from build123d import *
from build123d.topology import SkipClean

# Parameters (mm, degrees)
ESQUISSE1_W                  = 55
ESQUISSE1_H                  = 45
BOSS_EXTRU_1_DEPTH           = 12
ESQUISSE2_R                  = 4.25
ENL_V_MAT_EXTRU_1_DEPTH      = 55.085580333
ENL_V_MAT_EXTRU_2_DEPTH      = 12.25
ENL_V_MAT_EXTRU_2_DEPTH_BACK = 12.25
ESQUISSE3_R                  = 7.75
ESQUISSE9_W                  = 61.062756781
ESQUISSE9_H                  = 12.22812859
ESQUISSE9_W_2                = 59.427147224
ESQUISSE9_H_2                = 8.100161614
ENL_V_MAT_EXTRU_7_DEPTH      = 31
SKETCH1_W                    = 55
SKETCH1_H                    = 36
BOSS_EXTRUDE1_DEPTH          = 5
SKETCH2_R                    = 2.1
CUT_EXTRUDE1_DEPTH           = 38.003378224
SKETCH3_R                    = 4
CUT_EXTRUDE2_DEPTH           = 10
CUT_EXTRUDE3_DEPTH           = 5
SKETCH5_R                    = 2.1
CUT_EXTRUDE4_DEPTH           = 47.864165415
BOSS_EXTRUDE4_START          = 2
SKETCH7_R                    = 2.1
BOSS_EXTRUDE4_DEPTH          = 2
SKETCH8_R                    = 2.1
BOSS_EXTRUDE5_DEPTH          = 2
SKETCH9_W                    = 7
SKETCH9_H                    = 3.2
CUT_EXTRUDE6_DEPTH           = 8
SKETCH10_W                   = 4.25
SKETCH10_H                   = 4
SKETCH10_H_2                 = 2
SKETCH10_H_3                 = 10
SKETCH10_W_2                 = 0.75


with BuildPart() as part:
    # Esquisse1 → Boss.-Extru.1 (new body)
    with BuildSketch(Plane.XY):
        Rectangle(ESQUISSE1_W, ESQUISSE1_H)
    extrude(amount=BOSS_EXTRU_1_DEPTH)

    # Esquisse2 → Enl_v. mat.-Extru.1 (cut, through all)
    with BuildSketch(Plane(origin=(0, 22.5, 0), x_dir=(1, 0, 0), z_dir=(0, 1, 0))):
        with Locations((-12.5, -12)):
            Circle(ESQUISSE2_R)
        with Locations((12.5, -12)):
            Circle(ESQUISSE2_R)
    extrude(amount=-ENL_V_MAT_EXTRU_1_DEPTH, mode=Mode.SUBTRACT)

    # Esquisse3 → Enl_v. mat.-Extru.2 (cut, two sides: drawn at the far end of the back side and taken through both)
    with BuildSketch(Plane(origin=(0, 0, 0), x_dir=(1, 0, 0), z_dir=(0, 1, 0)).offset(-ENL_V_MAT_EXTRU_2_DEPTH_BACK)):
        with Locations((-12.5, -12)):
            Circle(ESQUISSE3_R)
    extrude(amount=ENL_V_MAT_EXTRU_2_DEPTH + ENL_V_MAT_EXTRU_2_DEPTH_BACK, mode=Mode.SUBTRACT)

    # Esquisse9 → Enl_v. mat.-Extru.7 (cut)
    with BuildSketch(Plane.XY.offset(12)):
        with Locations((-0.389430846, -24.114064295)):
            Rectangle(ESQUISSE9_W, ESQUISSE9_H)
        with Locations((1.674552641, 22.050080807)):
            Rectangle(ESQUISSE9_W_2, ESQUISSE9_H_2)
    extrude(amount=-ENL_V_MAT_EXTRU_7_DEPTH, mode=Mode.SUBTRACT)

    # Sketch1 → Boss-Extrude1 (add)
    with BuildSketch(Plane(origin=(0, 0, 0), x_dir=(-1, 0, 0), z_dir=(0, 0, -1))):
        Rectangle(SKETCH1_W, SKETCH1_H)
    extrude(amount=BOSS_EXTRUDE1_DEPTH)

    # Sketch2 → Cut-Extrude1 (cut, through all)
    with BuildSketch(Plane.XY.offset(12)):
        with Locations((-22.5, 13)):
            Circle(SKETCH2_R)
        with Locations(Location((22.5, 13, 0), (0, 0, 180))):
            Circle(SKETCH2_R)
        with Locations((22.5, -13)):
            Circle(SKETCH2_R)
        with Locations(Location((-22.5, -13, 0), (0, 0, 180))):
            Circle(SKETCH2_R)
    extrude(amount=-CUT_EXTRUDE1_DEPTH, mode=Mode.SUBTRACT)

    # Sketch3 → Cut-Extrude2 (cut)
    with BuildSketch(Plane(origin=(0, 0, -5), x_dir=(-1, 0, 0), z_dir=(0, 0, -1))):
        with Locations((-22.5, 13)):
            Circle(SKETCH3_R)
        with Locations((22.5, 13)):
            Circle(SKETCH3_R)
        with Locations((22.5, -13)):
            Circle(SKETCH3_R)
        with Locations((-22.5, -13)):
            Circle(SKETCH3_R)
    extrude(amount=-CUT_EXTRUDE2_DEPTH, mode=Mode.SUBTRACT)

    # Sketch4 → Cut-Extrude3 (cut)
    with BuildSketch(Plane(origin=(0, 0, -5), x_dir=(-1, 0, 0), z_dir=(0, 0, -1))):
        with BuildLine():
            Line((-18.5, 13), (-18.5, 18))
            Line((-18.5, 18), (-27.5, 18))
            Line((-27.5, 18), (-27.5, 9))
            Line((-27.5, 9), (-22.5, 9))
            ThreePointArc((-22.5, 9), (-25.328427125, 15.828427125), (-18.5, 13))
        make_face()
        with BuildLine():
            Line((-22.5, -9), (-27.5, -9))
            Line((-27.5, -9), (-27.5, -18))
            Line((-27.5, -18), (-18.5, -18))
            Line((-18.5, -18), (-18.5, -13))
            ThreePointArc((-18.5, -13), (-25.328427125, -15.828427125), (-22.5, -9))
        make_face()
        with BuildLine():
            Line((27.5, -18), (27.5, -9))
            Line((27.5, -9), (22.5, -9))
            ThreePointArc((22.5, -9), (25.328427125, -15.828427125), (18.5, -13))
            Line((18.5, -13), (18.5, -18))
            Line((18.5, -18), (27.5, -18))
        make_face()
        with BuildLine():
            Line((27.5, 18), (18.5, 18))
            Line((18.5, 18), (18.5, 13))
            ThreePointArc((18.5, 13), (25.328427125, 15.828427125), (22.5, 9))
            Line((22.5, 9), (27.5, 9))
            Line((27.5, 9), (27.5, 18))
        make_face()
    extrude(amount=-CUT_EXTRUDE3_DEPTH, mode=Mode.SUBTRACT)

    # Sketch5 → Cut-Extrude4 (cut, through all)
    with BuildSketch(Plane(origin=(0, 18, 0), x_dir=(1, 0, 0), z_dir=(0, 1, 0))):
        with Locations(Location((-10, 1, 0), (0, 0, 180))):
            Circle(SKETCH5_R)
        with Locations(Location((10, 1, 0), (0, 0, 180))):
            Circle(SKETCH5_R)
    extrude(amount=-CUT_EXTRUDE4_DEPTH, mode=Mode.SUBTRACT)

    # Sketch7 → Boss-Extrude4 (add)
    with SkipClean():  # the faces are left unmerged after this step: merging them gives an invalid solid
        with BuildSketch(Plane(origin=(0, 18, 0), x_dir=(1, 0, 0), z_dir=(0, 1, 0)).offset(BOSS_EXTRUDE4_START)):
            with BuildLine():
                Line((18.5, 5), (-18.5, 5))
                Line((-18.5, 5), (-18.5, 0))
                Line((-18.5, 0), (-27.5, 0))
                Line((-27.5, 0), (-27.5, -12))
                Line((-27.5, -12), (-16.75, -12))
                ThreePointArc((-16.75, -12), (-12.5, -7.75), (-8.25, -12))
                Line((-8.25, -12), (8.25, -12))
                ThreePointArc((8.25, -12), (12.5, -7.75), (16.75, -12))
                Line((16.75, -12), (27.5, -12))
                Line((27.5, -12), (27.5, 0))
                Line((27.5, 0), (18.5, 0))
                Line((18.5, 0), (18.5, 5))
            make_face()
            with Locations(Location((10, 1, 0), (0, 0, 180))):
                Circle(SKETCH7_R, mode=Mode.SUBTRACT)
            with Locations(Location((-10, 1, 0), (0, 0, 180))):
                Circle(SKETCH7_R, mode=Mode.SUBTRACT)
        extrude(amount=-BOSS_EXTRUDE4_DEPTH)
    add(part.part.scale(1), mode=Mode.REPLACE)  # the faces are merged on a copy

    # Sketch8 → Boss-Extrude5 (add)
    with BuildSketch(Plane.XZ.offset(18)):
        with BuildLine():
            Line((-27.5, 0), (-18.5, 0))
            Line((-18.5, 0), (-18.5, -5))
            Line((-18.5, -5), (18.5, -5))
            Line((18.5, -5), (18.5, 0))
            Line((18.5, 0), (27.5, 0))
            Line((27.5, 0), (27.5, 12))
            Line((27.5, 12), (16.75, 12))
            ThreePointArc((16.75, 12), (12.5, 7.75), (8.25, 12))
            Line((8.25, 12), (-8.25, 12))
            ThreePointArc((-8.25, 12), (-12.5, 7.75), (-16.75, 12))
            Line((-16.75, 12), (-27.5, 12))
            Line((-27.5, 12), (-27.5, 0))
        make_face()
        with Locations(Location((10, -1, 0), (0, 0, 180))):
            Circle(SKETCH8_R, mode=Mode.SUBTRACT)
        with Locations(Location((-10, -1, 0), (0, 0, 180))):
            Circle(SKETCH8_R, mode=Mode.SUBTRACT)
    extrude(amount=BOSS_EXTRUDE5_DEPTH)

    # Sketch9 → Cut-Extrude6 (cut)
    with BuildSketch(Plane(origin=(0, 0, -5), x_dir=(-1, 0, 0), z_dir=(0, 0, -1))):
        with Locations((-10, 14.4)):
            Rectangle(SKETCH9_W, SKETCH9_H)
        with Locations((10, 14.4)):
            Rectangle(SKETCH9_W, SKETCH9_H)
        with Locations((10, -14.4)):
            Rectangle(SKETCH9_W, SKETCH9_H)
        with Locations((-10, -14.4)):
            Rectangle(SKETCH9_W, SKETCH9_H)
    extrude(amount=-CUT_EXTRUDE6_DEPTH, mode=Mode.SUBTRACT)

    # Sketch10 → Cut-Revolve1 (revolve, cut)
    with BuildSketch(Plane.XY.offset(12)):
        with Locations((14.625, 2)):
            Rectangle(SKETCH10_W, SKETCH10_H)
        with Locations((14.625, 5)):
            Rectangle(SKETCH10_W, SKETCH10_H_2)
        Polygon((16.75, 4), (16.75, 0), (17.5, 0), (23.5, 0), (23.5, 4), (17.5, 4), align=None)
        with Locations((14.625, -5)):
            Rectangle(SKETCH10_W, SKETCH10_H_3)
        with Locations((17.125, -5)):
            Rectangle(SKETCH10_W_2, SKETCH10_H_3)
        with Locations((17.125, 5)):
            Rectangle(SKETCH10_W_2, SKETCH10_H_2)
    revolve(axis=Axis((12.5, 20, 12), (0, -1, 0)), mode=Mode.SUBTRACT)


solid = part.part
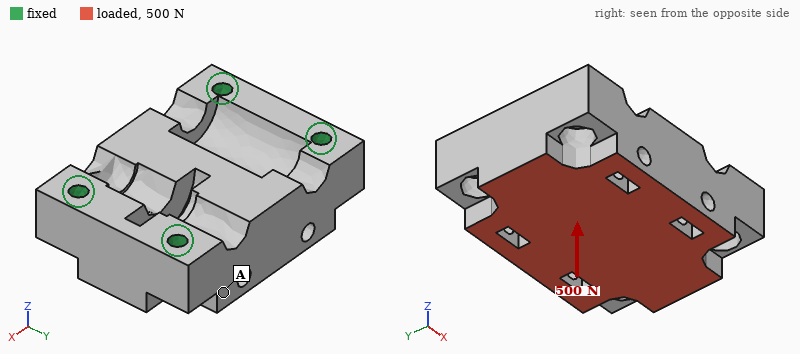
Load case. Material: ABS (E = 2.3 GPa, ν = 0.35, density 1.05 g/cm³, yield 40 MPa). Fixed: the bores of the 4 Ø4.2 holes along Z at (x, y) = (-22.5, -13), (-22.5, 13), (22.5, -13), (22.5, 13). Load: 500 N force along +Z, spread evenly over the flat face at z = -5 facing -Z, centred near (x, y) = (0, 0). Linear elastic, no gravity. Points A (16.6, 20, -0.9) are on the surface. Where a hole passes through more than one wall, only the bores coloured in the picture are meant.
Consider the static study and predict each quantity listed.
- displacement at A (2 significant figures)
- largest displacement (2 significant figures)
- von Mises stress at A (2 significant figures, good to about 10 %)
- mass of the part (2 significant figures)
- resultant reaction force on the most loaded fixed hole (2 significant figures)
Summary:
11 µm
24 µm
0.95 MPa
29 g
150 N
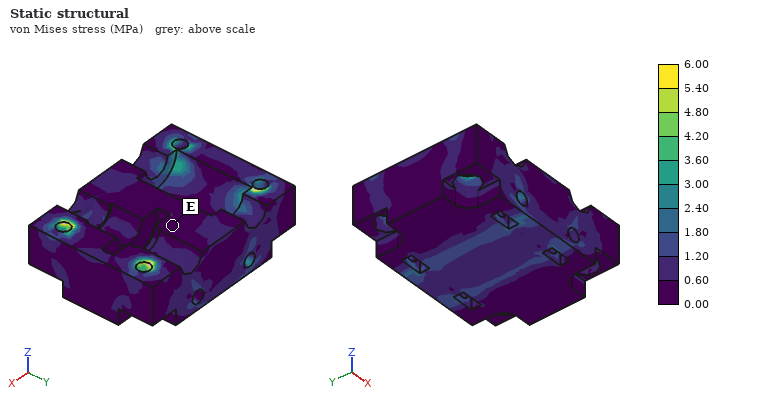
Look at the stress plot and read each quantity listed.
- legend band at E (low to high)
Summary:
0.00 to 0.60 MPa
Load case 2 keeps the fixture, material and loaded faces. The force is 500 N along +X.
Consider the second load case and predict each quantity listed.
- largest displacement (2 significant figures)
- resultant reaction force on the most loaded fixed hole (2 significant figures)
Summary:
22 µm
160 N
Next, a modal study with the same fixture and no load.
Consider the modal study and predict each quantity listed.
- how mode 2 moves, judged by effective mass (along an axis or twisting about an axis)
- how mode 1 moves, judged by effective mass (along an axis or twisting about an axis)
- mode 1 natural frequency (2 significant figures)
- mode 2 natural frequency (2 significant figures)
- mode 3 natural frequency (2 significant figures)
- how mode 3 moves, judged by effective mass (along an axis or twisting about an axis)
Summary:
along Y
along Z
4900 Hz
5500 Hz
5700 Hz
along Y
